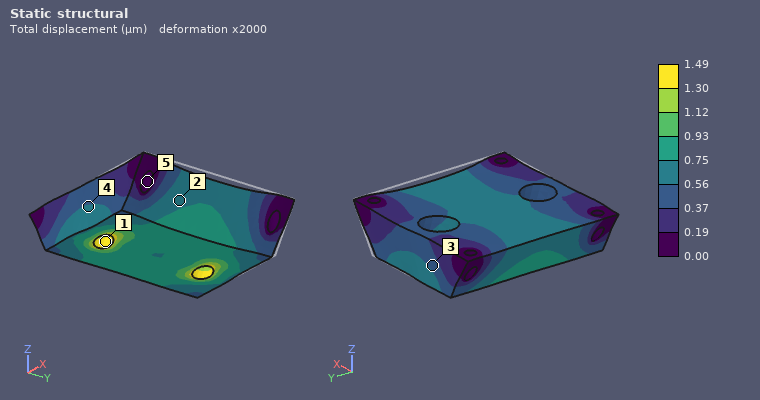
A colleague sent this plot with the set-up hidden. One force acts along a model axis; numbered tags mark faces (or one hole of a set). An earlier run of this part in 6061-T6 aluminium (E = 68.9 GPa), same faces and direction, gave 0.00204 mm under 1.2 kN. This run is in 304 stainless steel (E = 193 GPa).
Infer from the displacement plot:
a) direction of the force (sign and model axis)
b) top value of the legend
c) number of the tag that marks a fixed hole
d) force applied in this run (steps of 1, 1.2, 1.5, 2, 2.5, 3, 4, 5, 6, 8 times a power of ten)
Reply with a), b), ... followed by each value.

a) -X
b) 1.49 µm
c) 5
d) 2.5 kN
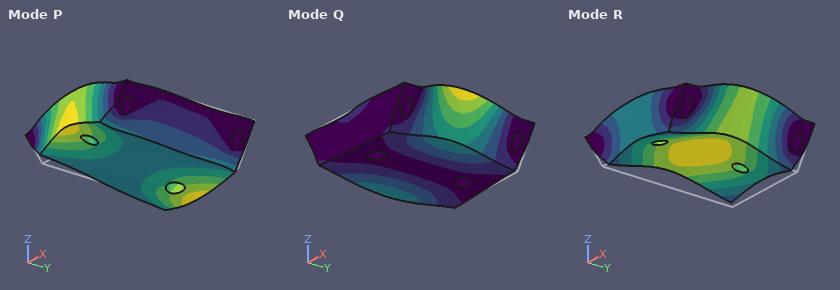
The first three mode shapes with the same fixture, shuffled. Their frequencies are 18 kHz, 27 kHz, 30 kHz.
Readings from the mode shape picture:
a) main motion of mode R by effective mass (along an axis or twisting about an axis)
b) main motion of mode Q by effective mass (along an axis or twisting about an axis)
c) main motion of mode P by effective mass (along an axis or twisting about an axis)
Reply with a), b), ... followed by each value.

a) along Z
b) along X
c) along Y
